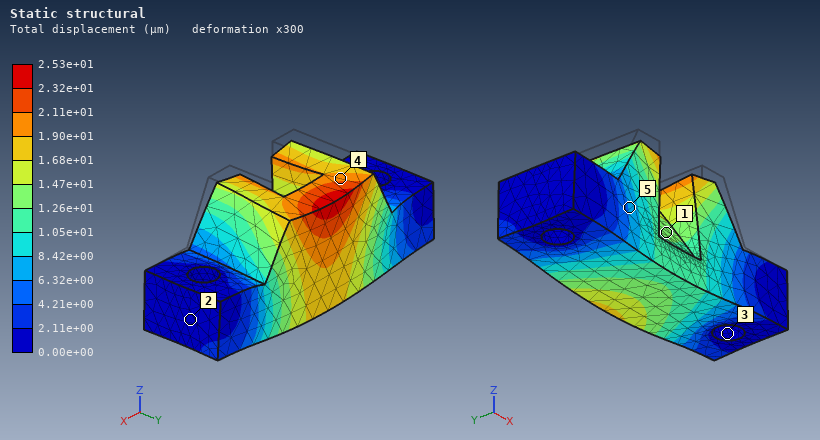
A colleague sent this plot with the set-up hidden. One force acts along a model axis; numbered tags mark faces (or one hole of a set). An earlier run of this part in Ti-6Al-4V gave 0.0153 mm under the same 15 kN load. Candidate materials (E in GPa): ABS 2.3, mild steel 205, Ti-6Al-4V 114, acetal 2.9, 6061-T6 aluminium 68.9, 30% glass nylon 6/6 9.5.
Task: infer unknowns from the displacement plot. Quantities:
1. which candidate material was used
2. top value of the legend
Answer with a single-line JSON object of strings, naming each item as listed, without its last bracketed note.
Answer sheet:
{"which candidate material was used": "6061-T6 aluminium", "top value of the legend": "2.53e+01 µm"}
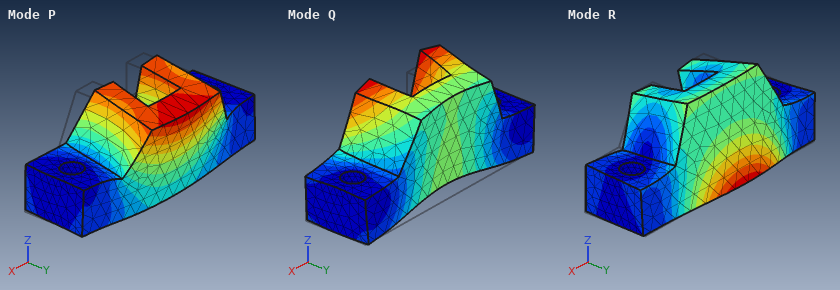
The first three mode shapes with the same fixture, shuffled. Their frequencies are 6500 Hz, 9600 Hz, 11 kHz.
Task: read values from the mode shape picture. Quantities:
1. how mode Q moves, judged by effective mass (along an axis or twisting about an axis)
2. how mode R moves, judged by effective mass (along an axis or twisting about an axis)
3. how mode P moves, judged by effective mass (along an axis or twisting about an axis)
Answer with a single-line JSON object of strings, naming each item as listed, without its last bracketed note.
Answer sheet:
{"how mode Q moves, judged by effective mass": "along Z", "how mode R moves, judged by effective mass": "along Y", "how mode P moves, judged by effective mass": "along Y"}
